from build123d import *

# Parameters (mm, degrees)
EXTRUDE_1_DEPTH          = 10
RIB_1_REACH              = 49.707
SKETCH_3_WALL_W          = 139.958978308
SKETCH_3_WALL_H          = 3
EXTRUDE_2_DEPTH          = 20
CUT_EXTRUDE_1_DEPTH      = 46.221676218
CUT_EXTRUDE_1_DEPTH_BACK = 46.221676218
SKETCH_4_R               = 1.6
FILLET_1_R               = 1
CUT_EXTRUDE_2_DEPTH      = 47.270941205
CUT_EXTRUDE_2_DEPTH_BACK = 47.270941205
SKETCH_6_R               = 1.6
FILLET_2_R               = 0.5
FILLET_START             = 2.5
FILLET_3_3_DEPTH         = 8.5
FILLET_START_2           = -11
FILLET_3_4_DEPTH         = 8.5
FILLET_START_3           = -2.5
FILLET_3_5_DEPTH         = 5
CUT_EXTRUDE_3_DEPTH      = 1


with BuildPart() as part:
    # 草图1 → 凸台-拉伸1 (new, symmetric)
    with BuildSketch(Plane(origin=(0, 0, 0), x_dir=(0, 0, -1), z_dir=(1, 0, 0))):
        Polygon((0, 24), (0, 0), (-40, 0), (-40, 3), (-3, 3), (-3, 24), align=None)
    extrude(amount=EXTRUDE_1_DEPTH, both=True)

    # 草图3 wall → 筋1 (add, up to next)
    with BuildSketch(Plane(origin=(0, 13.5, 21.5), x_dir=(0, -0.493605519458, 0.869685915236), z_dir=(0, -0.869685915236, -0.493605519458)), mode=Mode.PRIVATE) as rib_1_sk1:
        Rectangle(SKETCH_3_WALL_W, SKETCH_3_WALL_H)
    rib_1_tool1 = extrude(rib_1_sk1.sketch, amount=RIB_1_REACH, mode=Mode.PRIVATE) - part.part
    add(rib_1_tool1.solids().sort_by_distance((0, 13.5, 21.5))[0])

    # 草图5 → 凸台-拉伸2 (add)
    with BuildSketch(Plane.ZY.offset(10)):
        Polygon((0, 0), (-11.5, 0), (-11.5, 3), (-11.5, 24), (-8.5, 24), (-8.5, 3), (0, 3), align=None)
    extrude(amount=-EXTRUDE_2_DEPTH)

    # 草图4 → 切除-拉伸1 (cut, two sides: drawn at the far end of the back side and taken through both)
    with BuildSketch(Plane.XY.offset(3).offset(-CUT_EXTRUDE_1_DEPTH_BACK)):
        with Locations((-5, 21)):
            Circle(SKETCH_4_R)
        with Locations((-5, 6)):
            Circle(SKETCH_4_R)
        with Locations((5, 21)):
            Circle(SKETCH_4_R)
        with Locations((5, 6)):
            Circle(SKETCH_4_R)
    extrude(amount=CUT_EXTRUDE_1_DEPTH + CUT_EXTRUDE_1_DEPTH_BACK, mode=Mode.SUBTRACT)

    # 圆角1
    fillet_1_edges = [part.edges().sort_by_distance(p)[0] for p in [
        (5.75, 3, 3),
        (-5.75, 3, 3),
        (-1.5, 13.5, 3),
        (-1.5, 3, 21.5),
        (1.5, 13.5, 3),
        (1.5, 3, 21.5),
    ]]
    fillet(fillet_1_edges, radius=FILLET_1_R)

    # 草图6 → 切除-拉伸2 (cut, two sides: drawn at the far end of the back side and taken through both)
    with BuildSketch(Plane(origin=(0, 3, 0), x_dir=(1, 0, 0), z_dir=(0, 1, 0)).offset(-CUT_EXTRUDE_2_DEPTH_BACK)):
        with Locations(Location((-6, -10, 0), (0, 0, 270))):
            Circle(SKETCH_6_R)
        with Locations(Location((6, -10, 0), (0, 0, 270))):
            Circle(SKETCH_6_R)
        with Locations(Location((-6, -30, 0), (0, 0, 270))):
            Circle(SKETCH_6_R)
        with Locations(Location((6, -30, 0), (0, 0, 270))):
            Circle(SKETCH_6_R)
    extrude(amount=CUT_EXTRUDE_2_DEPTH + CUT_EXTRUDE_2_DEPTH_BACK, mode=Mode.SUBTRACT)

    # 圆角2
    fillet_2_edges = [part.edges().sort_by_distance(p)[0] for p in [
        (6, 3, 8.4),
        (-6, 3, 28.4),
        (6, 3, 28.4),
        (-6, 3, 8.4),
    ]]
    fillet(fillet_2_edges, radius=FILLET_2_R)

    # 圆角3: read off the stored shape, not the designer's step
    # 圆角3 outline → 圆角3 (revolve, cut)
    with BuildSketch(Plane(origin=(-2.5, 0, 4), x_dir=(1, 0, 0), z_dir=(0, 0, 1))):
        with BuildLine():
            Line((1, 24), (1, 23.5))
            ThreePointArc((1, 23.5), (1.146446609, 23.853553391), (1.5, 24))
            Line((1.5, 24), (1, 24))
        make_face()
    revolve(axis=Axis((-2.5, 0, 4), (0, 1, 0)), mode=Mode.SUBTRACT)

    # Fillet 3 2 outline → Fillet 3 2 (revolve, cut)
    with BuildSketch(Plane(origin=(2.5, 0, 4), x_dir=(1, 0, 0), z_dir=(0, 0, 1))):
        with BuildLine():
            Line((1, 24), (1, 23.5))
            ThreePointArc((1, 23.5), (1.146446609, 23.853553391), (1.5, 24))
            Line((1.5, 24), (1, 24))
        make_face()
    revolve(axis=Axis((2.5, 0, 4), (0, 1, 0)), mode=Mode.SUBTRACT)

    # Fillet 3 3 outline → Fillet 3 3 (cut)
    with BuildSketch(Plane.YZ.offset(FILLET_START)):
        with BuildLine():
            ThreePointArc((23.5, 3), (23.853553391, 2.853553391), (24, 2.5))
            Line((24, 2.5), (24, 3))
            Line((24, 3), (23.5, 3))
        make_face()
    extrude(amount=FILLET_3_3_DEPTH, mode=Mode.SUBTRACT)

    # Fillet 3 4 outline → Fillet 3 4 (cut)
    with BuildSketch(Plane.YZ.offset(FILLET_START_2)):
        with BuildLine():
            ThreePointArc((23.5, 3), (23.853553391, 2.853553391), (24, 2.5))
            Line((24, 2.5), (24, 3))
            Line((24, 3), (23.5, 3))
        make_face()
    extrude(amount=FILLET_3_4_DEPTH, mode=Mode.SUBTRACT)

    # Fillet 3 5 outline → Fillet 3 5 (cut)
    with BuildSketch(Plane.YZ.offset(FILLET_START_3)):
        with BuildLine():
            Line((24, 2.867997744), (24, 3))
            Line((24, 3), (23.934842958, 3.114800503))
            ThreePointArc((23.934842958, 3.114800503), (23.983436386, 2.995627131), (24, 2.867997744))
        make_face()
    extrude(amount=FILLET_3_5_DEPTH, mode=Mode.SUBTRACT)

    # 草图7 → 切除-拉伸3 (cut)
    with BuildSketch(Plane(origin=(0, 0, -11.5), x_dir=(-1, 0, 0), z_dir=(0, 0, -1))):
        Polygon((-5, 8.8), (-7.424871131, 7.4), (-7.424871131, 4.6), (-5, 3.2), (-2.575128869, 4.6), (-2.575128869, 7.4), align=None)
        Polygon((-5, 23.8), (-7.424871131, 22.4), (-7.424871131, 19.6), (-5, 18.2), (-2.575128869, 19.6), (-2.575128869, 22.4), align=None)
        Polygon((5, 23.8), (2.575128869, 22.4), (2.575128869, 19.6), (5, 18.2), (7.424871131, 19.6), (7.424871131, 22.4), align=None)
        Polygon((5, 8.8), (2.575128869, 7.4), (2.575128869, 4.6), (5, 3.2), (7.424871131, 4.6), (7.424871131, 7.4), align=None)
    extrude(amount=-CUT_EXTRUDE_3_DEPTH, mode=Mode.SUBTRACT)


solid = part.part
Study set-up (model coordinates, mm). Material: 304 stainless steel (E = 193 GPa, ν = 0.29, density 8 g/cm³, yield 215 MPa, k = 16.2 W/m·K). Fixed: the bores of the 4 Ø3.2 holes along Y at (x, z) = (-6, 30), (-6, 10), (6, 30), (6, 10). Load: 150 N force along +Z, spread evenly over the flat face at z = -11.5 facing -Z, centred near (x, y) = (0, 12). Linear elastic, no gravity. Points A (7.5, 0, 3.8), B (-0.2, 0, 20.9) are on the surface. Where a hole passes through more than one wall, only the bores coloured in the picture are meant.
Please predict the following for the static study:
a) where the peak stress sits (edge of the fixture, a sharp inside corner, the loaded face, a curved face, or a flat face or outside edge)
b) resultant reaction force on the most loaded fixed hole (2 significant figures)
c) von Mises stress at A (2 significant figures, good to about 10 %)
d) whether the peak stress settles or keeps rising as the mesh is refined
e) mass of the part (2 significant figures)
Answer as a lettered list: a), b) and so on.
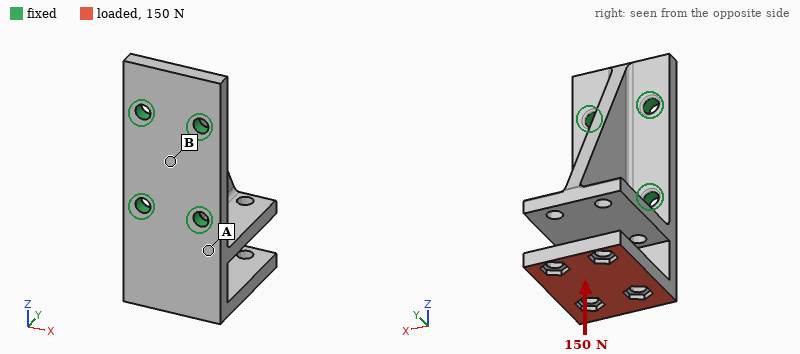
a) a sharp inside corner
b) 57 N
c) 13 MPa
d) keeps rising
e) 52 g
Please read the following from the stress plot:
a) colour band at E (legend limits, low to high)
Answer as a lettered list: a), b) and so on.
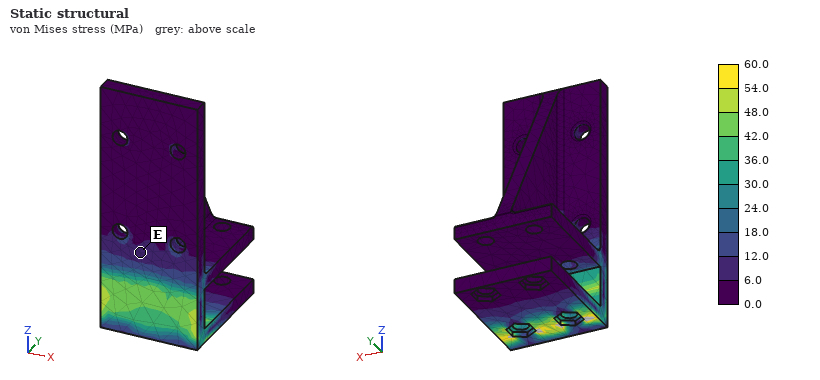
a) 6.0 to 12.0 MPa
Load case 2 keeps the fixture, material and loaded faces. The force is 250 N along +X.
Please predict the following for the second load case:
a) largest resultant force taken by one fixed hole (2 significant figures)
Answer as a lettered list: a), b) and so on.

a) 440 N
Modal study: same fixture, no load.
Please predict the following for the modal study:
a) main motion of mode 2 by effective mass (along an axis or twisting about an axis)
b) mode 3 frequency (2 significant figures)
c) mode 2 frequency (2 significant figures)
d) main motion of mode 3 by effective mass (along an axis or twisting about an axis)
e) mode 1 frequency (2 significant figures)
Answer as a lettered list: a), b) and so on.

a) along X
b) 6400 Hz
c) 4000 Hz
d) along Y
e) 2500 Hz
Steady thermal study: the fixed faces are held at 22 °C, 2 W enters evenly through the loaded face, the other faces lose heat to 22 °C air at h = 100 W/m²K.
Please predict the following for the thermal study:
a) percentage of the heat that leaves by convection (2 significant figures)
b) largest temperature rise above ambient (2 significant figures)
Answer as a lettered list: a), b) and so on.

a) 84 %
b) 17 K
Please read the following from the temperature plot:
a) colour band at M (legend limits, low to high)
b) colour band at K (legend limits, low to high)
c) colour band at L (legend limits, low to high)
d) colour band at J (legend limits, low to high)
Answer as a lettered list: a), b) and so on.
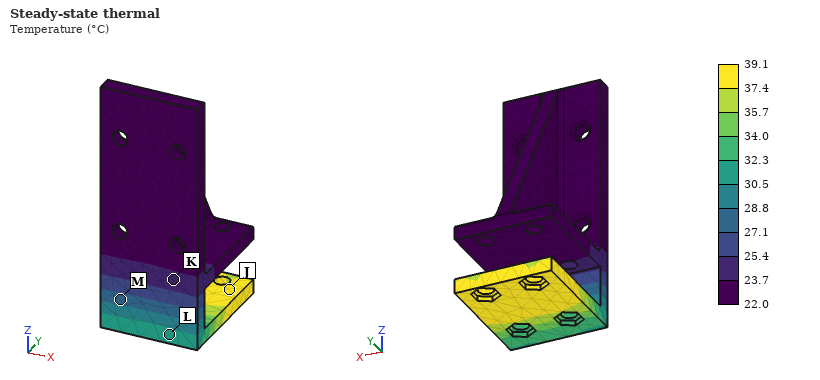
a) 27.1 to 28.8 °C
b) 23.7 to 25.4 °C
c) 30.5 to 32.3 °C
d) 37.4 to 39.1 °C
